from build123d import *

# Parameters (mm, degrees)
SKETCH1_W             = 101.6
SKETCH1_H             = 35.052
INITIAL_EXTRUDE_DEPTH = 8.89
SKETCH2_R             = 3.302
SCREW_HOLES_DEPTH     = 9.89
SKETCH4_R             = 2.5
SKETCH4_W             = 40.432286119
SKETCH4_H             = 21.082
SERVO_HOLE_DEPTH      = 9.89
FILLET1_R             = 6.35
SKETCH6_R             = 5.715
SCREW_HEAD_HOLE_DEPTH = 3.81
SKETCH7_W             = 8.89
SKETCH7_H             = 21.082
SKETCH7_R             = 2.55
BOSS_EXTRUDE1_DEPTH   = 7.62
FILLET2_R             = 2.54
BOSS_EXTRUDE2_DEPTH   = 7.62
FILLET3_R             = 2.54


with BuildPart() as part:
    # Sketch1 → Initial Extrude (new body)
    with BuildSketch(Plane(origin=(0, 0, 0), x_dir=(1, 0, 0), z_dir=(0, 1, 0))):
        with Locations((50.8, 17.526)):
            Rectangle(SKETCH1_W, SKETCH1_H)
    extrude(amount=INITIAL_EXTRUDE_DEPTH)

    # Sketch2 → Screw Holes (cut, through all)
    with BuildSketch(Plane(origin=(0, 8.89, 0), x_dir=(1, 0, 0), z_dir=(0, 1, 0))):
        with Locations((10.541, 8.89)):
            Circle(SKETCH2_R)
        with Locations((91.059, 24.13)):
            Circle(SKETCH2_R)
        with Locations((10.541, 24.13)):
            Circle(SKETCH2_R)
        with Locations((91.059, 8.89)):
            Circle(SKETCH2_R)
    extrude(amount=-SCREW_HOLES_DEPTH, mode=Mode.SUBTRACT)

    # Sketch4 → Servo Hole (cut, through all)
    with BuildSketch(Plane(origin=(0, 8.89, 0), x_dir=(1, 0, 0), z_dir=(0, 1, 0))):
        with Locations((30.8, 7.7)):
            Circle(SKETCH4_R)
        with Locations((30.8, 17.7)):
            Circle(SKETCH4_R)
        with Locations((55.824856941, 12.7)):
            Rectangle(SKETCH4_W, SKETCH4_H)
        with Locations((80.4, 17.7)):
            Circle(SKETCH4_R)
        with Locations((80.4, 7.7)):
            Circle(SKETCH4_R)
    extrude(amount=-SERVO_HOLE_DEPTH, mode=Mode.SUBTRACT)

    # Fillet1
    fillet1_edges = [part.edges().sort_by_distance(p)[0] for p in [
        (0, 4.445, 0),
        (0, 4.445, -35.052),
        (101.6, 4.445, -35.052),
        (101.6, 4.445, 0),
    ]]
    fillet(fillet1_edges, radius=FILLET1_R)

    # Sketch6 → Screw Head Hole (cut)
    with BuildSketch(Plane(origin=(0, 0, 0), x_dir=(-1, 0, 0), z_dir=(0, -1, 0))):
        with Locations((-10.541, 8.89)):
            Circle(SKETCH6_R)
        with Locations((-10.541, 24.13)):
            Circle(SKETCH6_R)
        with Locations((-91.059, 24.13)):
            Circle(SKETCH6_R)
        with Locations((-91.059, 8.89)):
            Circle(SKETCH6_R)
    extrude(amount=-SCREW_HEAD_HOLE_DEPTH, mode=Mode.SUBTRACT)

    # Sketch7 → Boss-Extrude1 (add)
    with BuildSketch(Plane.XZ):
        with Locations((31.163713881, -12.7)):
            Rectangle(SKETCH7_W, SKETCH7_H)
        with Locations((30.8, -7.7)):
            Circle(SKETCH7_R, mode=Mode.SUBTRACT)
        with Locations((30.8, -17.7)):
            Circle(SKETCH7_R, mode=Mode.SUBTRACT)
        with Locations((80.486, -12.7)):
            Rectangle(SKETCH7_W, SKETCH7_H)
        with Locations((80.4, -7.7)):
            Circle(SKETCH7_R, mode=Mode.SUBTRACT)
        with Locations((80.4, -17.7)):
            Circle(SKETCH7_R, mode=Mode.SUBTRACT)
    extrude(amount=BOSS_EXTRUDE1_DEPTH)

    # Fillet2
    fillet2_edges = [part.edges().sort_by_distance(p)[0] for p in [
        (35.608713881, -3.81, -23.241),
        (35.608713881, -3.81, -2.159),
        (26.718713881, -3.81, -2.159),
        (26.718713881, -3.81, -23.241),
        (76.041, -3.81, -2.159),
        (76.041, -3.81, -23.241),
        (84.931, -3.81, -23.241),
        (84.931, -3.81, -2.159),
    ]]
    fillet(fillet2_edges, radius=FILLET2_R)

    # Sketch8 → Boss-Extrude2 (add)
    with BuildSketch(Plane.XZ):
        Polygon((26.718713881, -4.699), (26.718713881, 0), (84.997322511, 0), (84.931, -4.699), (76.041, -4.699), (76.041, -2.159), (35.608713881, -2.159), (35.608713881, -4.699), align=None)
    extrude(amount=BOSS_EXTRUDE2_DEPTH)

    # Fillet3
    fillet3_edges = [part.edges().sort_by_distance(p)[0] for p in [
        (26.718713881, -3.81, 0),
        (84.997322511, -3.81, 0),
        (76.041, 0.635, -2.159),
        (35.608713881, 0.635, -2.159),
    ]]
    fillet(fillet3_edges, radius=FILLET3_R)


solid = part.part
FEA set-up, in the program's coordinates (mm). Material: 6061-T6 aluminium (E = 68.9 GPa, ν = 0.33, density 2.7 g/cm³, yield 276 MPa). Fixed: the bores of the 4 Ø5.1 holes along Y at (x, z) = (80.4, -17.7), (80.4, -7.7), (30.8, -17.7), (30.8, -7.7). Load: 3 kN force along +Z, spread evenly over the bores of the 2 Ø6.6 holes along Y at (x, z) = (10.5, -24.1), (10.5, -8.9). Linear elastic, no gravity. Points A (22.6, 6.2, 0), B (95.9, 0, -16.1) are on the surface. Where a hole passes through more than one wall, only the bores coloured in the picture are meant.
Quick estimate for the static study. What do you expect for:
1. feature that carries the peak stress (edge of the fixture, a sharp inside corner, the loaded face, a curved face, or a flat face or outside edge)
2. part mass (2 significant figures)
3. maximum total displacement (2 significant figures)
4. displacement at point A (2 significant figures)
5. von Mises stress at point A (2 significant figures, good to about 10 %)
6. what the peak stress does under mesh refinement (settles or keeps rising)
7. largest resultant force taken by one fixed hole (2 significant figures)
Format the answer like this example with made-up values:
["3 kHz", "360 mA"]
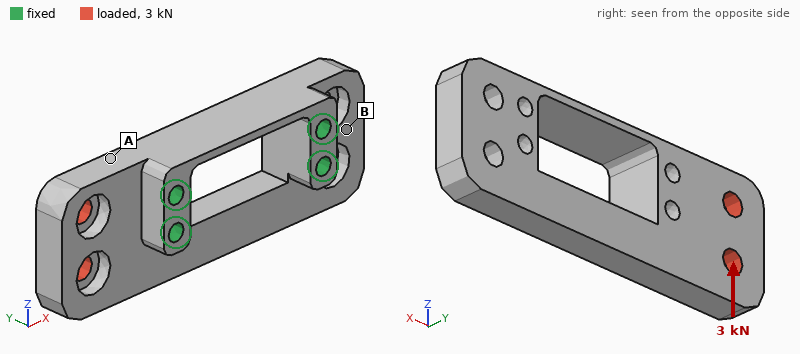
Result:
["edge of the fixture", "65 g", "57 µm", "22 µm", "26 MPa", "keeps rising", "3.3 kN"]
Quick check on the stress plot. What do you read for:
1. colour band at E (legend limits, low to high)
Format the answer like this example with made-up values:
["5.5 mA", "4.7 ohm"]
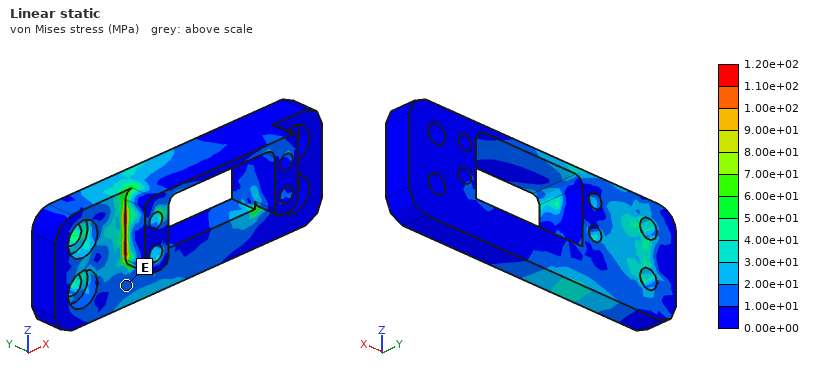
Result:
["1.00e+01 to 2.00e+01 MPa"]
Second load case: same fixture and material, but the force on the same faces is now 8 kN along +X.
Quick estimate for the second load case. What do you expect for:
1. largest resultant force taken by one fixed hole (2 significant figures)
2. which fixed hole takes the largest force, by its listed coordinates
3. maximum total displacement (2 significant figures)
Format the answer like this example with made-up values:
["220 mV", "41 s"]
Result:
["3.5 kN", "(30.8, -17.7)", "0.15 mm"]
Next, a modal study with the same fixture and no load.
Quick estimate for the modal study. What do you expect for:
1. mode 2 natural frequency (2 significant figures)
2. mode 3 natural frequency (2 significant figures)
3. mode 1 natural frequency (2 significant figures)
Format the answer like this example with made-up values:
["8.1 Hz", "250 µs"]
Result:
["7000 Hz", "8800 Hz", "5700 Hz"]
